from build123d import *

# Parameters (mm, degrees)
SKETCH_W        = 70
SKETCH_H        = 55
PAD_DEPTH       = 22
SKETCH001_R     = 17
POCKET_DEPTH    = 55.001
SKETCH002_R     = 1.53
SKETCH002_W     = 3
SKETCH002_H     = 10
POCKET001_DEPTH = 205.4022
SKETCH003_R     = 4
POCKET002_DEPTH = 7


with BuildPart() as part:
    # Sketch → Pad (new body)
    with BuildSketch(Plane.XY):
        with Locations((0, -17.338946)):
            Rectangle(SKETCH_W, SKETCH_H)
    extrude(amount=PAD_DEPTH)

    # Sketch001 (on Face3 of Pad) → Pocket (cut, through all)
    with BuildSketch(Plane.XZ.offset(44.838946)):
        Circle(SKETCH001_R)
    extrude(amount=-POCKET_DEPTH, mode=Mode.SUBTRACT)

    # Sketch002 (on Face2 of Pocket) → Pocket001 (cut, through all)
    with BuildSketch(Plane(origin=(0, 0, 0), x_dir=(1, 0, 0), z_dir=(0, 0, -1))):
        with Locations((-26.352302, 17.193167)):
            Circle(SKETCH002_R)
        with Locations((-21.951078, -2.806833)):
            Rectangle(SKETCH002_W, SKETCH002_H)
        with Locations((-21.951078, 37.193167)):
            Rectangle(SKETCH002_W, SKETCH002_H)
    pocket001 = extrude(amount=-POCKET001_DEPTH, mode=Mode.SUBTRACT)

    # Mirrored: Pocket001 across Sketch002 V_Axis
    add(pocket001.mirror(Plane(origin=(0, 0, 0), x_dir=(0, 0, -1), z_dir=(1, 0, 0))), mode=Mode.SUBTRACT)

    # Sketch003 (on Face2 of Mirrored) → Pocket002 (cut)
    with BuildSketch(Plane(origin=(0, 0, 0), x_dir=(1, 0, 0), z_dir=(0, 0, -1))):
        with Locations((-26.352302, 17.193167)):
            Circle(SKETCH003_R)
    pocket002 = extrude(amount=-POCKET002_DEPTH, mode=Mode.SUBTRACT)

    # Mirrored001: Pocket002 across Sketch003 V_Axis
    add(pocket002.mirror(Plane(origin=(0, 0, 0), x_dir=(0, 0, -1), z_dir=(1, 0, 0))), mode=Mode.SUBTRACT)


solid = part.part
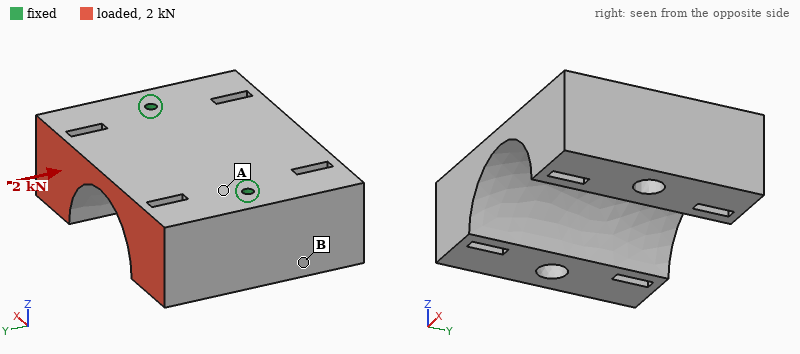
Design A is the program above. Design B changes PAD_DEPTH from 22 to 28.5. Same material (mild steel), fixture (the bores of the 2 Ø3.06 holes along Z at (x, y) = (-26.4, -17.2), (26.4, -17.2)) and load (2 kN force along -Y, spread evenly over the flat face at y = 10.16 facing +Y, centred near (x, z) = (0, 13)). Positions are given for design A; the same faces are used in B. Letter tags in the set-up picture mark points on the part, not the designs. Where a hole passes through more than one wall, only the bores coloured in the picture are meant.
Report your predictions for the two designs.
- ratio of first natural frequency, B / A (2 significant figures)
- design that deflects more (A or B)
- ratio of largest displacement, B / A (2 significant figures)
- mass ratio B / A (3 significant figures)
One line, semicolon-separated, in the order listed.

1.3; A; 0.55; 1.43
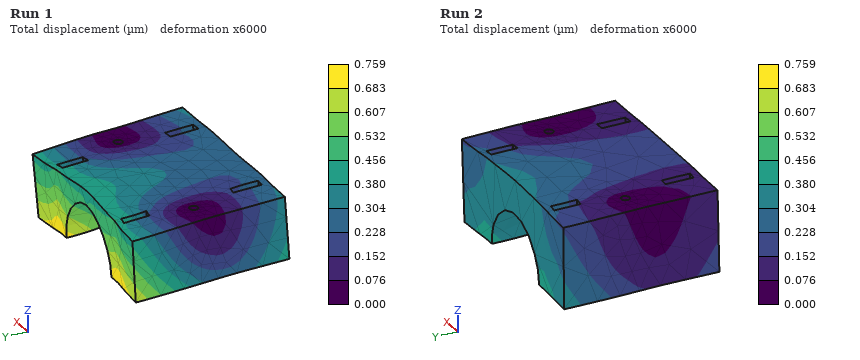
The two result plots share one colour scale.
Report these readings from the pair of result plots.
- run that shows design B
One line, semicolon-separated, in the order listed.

Run 2
